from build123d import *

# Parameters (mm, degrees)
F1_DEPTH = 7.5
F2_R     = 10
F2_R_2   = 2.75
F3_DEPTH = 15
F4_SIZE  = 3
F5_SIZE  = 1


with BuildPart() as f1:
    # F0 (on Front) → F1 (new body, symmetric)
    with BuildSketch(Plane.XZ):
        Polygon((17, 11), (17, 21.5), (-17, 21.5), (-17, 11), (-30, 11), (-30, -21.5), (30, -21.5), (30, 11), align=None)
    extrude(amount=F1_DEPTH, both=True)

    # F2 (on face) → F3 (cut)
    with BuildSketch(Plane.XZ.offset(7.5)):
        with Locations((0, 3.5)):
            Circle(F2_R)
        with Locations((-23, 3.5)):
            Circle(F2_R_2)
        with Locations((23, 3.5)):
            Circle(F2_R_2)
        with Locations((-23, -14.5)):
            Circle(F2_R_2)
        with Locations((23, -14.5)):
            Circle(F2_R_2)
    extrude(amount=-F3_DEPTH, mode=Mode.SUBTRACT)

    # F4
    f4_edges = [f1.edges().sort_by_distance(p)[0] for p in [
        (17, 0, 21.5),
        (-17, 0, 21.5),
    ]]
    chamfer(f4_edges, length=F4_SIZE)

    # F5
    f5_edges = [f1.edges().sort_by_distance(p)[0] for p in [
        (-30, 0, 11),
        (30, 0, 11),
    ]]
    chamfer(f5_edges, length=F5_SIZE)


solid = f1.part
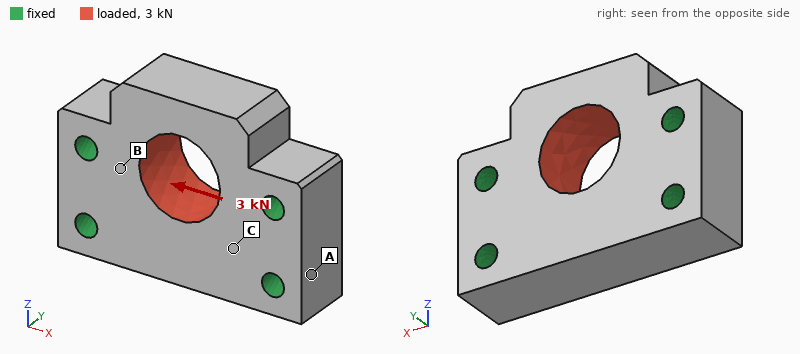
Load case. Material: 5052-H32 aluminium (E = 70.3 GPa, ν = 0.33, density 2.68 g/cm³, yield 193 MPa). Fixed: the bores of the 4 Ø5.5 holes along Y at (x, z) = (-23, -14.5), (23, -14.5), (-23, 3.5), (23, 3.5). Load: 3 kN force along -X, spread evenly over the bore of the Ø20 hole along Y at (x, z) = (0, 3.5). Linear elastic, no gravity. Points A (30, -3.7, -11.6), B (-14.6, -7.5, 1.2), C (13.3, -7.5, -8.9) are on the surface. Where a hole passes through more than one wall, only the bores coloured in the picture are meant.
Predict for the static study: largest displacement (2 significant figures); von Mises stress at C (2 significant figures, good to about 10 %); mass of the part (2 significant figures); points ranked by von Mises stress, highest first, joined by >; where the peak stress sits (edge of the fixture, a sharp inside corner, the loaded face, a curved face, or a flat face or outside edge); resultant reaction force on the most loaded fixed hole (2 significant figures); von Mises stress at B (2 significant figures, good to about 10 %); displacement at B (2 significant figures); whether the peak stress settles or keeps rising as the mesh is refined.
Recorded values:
2.4 µm
2.2 MPa
76 g
B > C > A
edge of the fixture
1.1 kN
3.6 MPa
0.40 µm
keeps rising
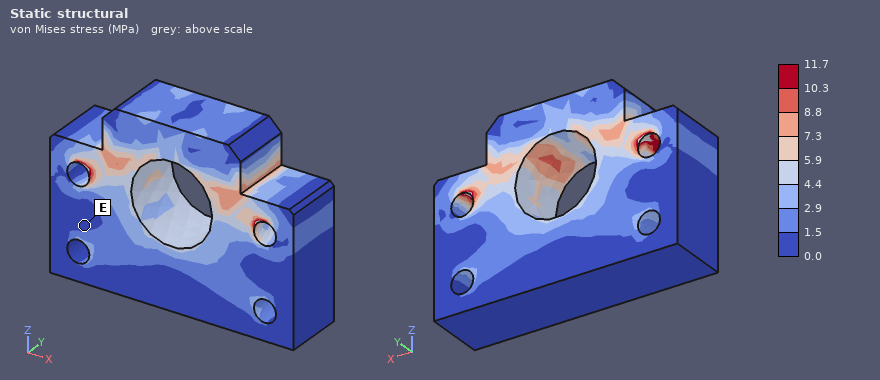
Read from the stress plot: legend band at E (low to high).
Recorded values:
0.0 to 1.5 MPa
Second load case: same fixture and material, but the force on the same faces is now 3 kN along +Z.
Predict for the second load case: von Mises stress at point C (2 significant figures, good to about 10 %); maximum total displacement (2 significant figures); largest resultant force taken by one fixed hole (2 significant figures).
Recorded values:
5.0 MPa
3.2 µm
920 N
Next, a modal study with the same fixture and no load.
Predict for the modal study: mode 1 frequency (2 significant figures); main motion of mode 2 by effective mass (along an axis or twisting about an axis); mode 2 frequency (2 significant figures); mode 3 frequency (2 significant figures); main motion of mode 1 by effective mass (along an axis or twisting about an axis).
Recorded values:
17 kHz
along Y
27 kHz
30 kHz
along Y
